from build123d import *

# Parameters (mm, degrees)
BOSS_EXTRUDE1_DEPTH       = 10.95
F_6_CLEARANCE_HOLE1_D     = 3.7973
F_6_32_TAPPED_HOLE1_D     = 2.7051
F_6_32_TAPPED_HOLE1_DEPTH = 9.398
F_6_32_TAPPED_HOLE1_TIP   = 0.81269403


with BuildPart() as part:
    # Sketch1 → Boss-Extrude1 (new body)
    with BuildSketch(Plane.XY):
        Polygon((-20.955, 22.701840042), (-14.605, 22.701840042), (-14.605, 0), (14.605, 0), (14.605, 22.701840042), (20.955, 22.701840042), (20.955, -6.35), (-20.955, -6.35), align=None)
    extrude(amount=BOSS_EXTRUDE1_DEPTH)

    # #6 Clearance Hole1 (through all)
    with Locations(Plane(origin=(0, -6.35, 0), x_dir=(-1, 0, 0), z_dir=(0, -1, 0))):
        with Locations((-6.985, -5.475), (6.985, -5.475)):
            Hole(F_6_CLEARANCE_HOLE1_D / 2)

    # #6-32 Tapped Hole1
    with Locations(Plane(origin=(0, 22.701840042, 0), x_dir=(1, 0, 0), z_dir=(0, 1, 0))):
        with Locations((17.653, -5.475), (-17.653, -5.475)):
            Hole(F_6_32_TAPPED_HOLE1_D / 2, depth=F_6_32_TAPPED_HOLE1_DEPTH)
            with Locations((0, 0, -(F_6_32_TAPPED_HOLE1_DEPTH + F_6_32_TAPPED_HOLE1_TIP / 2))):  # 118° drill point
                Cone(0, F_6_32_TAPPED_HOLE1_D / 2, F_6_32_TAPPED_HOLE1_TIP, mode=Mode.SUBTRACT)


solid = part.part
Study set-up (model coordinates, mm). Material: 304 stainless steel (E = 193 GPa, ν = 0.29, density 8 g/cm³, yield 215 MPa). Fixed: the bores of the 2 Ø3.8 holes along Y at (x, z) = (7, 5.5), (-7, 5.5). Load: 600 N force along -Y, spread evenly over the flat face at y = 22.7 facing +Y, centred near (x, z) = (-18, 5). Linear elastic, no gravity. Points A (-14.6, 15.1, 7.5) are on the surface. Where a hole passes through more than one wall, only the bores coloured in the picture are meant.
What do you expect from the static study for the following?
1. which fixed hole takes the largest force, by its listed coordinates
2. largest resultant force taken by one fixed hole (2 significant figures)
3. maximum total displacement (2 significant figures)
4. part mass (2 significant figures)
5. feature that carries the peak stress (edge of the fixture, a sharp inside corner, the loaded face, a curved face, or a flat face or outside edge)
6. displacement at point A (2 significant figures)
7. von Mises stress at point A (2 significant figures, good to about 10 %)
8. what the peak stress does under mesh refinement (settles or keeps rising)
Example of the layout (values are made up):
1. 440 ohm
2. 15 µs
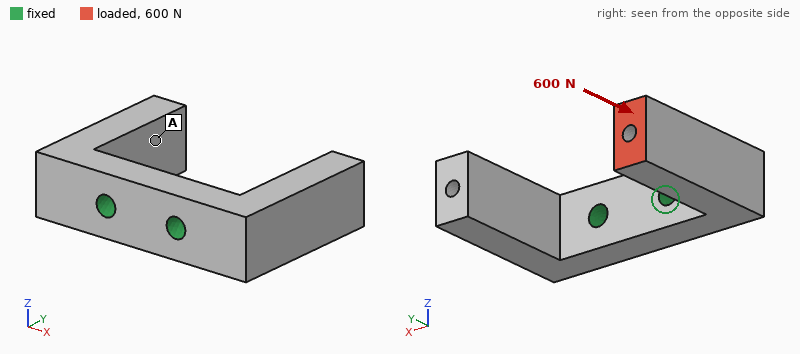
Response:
1. (-7, 5.5)
2. 660 N
3. 22 µm
4. 47 g
5. edge of the fixture
6. 14 µm
7. 9.3 MPa
8. keeps rising
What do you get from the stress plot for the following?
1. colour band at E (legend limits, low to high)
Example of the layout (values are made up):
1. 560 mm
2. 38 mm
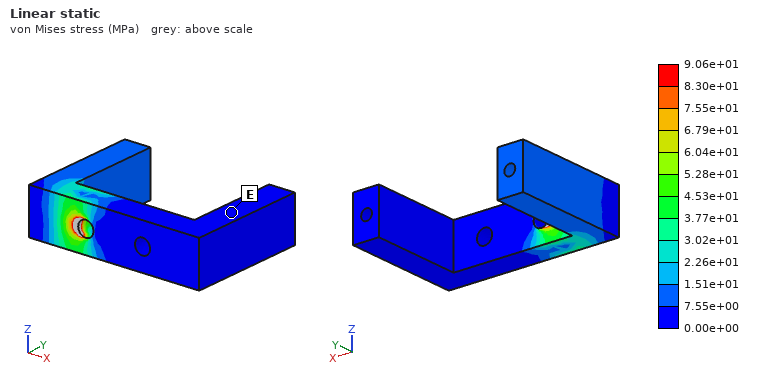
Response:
1. 0.00e+00 to 7.55e+00 MPa
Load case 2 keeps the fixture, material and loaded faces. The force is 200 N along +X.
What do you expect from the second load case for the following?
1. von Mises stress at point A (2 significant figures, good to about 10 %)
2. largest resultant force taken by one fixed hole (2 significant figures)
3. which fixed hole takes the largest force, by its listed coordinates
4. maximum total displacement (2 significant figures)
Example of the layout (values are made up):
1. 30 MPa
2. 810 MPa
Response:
1. 21 MPa
2. 190 N
3. (-7, 5.5)
4. 53 µm
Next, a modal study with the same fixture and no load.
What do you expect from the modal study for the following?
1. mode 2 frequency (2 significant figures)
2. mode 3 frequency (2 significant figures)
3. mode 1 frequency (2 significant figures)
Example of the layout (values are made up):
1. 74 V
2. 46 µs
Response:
1. 4900 Hz
2. 5800 Hz
3. 4900 Hz
